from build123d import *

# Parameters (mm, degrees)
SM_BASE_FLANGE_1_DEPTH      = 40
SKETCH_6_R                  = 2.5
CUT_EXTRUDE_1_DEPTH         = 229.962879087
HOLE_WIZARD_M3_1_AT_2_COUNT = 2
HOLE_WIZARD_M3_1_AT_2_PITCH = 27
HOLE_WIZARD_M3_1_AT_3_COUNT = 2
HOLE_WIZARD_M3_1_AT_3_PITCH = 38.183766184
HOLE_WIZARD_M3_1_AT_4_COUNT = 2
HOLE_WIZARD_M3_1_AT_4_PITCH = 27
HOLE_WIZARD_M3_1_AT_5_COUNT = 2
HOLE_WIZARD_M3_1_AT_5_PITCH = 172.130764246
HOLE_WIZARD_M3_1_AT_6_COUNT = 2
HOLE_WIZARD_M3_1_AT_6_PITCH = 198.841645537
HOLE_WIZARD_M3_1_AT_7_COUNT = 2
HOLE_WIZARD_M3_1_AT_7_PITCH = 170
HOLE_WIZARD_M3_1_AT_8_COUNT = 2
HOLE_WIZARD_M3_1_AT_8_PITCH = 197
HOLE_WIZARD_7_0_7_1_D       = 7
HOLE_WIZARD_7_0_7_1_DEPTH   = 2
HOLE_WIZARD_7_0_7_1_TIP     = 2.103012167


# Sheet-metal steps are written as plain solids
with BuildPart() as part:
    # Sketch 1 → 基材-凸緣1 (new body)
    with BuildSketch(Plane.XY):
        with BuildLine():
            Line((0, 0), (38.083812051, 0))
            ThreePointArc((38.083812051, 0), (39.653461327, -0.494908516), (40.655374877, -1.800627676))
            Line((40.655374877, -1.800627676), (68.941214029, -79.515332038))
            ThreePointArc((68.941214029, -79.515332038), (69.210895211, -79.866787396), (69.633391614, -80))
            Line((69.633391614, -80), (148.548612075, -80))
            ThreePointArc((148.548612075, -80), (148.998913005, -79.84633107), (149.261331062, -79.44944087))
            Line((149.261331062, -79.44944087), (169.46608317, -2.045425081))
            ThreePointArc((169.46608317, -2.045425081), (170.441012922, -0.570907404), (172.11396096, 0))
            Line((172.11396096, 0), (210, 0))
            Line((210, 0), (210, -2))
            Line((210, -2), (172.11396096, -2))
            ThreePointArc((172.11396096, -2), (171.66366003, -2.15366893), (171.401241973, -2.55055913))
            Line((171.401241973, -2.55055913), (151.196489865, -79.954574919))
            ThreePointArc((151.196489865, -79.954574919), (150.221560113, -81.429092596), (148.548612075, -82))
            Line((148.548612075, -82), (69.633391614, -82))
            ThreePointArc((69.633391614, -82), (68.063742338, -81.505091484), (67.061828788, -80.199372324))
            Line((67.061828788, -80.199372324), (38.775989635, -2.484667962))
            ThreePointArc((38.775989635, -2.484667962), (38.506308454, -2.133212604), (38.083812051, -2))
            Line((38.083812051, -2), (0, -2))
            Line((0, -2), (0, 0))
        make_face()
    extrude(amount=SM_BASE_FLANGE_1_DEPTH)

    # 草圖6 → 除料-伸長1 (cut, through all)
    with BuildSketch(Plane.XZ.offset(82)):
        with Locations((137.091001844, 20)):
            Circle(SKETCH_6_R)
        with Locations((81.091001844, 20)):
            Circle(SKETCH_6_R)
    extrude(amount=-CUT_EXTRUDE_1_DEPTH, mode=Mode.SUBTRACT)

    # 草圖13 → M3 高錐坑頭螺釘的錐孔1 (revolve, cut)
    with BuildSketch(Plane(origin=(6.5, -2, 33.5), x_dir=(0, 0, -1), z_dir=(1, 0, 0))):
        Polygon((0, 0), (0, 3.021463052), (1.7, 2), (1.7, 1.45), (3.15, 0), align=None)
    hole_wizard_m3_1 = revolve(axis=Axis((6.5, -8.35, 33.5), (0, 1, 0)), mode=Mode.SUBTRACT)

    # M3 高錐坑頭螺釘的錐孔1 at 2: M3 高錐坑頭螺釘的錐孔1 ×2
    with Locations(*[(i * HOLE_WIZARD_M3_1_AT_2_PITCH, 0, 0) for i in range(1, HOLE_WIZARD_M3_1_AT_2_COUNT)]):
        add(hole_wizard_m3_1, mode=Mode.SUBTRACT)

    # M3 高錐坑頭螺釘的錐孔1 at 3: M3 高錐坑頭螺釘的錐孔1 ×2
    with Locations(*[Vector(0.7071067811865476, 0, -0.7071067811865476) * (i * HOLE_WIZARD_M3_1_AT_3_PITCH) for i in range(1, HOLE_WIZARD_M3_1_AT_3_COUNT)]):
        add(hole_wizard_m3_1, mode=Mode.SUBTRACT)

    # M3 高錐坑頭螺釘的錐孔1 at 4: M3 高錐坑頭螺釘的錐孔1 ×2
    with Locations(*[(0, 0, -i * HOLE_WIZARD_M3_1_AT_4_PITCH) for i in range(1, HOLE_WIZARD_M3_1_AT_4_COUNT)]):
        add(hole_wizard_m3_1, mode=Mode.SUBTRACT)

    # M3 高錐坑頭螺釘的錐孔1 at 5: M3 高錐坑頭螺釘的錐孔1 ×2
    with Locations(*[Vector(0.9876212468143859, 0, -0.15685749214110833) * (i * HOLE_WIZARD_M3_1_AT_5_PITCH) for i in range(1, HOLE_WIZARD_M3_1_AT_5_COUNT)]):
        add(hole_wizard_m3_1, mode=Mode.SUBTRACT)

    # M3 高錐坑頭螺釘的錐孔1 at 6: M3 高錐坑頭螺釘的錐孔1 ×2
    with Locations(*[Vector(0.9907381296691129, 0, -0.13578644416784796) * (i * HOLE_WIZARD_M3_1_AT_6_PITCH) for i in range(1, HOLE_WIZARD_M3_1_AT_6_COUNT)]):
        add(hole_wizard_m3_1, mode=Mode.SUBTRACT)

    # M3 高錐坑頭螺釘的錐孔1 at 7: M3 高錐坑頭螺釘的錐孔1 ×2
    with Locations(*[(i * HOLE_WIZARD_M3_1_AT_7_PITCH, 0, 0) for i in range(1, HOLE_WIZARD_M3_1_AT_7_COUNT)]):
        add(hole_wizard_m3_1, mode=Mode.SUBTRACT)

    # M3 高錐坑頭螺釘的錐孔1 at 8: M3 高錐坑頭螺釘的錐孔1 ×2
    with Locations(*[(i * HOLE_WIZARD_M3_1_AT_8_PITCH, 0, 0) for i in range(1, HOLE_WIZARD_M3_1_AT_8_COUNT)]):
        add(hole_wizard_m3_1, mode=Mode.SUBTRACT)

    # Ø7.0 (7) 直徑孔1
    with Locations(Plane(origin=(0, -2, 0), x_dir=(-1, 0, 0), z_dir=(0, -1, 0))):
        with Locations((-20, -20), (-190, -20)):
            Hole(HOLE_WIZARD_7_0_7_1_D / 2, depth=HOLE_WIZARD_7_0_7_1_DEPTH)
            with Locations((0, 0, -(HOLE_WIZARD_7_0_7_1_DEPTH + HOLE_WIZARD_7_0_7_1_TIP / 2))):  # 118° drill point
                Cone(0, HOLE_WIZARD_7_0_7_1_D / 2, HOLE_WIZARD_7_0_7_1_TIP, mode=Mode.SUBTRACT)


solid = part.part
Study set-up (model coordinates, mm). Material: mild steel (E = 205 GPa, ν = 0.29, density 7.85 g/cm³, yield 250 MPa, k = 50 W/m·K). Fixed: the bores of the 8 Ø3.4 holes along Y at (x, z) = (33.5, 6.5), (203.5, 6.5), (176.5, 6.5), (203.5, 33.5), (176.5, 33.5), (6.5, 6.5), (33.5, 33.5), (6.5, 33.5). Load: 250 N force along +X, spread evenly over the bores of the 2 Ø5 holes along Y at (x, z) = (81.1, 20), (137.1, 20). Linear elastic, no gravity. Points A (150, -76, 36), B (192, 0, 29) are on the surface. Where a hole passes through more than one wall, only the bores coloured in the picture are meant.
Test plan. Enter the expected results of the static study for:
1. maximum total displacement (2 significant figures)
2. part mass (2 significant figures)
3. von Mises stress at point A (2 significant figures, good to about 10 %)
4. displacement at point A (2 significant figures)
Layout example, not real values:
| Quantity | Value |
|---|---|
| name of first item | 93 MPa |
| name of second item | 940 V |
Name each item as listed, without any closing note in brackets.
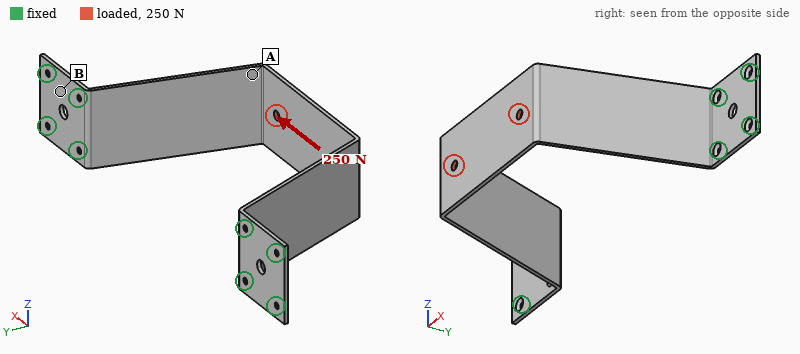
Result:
| Quantity | Value |
|---|---|
| maximum total displacement | 1.1 mm |
| part mass | 200 g |
| von Mises stress at point A | 120 MPa |
| displacement at point A | 1.0 mm |
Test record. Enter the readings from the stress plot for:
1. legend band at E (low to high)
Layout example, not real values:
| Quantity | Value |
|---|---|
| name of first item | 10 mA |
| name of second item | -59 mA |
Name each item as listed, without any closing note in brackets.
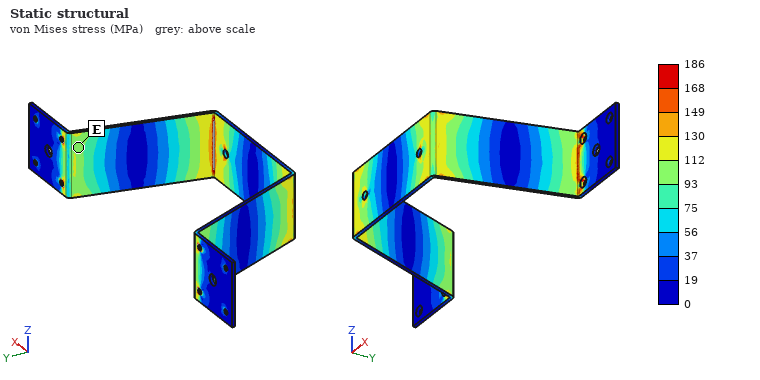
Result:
| Quantity | Value |
|---|---|
| legend band at E | 93 to 112 MPa |
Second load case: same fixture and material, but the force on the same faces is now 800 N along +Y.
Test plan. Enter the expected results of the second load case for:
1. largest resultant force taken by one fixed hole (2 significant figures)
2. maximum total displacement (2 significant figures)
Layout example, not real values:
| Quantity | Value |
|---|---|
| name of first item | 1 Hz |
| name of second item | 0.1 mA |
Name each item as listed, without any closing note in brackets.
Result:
| Quantity | Value |
|---|---|
| largest resultant force taken by one fixed hole | 260 N |
| maximum total displacement | 0.36 mm |
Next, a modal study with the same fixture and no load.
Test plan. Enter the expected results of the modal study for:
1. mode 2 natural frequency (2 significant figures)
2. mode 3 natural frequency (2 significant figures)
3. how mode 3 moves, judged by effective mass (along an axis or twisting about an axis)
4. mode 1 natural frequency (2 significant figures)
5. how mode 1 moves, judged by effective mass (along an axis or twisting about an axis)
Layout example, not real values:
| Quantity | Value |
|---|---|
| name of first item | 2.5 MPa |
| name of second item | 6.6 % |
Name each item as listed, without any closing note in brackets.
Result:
| Quantity | Value |
|---|---|
| mode 2 natural frequency | 830 Hz |
| mode 3 natural frequency | 900 Hz |
| how mode 3 moves, judged by effective mass | along Z |
| mode 1 natural frequency | 250 Hz |
| how mode 1 moves, judged by effective mass | along X |
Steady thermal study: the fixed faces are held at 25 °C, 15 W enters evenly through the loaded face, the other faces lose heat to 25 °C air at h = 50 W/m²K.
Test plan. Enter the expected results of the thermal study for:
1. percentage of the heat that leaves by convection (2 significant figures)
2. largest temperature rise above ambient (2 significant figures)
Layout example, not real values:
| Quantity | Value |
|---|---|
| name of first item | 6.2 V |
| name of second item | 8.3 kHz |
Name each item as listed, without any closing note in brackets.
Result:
| Quantity | Value |
|---|---|
| percentage of the heat that leaves by convection | 96 % |
| largest temperature rise above ambient | 46 K |
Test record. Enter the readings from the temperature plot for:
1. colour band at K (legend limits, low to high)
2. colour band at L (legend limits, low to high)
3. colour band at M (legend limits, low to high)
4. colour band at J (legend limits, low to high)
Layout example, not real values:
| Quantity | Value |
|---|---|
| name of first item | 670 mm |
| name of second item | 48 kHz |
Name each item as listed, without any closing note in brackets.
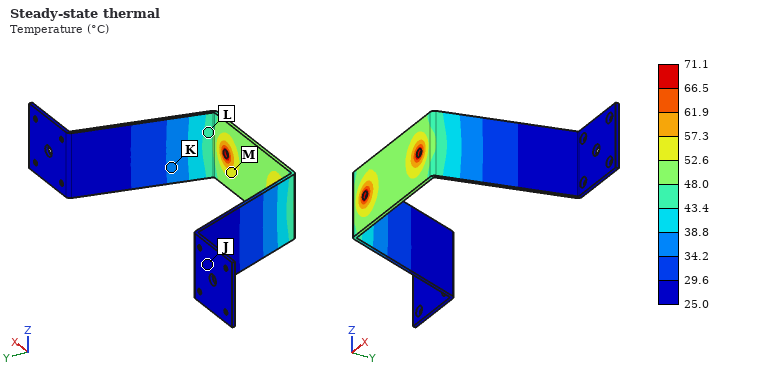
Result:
| Quantity | Value |
|---|---|
| colour band at K | 34.2 to 38.8 °C |
| colour band at L | 43.4 to 48.0 °C |
| colour band at M | 52.6 to 57.3 °C |
| colour band at J | 25.0 to 29.6 °C |
